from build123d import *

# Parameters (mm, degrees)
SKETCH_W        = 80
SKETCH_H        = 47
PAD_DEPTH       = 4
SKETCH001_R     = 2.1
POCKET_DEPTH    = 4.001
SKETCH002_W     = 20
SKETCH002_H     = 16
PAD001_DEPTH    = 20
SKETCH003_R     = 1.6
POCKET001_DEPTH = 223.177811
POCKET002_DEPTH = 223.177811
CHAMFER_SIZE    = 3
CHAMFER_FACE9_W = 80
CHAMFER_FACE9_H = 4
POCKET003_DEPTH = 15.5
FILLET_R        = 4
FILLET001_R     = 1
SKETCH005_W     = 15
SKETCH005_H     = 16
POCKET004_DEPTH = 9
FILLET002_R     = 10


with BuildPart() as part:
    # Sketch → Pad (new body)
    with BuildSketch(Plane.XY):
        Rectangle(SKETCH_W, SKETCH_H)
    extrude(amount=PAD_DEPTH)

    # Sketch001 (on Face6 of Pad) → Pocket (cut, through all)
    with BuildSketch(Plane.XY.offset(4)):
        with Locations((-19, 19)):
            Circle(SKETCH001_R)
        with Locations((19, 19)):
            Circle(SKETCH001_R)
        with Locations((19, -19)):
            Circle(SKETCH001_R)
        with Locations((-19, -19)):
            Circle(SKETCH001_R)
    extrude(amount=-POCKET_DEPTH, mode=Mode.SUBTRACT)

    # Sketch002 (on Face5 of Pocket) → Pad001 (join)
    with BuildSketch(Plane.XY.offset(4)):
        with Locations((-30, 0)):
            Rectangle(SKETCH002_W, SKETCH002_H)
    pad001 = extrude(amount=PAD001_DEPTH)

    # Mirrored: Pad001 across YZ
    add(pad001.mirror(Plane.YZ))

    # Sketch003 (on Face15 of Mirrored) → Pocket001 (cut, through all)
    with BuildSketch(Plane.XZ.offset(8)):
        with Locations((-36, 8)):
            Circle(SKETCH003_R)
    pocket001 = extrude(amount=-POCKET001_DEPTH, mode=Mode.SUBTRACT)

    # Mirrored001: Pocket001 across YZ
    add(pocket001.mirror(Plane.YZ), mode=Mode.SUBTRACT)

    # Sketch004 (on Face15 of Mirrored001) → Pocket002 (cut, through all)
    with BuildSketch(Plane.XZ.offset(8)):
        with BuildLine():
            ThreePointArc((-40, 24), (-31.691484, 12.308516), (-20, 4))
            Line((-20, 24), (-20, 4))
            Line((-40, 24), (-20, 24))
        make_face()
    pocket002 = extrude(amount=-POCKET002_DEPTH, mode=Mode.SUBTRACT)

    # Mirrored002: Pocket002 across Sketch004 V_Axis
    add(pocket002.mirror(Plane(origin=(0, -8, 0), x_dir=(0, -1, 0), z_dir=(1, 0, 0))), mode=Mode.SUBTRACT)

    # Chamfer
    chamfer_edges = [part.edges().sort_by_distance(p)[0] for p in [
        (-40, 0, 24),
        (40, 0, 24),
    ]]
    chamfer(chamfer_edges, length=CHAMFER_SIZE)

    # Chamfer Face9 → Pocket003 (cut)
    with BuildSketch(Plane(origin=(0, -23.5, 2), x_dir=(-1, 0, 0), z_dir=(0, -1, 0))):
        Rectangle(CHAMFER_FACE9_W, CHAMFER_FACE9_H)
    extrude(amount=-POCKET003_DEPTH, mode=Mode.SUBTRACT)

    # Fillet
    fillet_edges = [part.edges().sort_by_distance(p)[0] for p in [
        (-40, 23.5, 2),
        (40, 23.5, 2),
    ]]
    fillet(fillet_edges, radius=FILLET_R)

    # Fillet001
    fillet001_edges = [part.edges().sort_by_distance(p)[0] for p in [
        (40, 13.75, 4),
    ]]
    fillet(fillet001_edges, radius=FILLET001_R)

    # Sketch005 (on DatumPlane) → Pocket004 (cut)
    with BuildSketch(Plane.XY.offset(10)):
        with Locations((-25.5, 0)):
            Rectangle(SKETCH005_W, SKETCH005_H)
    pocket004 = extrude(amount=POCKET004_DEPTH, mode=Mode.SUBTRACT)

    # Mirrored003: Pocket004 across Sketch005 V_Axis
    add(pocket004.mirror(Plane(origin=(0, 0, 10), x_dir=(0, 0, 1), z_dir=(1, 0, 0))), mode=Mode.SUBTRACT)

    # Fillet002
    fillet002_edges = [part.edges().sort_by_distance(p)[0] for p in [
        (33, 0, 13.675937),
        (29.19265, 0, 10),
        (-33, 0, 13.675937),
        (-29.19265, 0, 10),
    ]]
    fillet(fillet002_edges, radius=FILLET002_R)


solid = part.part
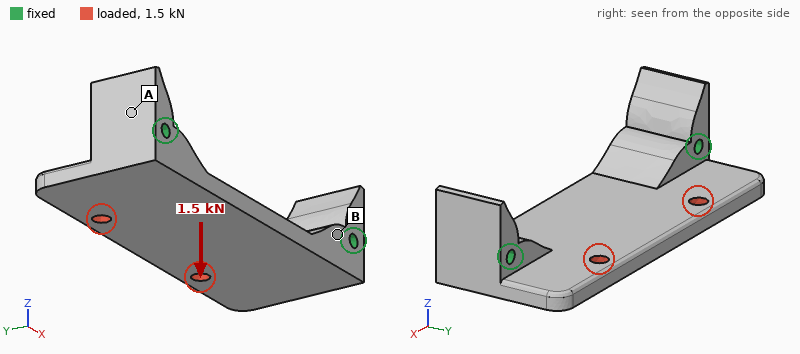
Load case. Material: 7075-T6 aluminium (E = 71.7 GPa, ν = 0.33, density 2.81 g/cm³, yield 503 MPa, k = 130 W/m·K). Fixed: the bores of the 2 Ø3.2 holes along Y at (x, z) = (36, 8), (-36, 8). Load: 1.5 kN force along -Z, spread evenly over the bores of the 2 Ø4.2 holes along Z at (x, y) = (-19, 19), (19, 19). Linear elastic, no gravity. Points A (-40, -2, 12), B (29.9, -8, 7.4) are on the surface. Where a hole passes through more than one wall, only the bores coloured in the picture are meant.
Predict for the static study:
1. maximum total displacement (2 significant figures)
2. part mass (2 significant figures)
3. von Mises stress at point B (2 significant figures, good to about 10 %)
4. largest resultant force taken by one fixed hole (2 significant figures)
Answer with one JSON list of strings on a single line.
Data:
["0.20 mm", "40 g", "23 MPa", "1.2 kN"]
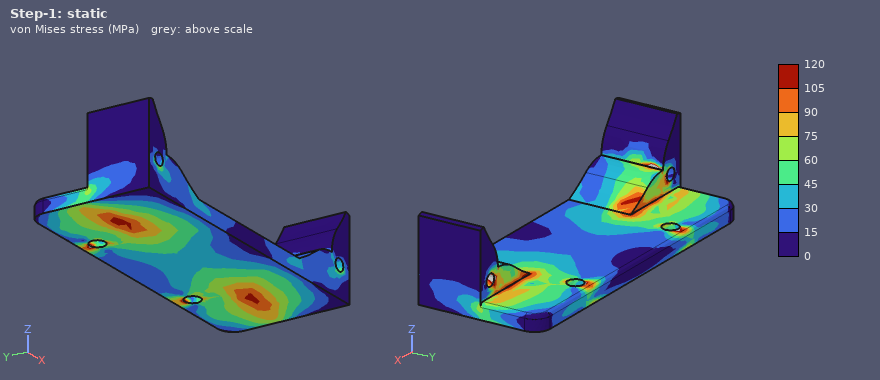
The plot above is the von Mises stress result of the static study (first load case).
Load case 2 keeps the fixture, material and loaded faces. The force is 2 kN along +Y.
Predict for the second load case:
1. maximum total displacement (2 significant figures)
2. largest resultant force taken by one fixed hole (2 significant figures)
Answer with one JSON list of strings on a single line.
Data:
["17 µm", "1.0 kN"]
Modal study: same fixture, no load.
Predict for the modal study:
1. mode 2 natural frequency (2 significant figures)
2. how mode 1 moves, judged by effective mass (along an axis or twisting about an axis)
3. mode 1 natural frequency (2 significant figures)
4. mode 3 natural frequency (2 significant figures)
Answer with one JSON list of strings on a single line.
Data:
["8700 Hz", "along Z", "5200 Hz", "9200 Hz"]
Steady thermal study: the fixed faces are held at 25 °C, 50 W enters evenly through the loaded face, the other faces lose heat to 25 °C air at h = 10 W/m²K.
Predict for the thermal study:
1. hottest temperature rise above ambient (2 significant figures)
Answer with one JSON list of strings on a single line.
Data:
["50 K"]
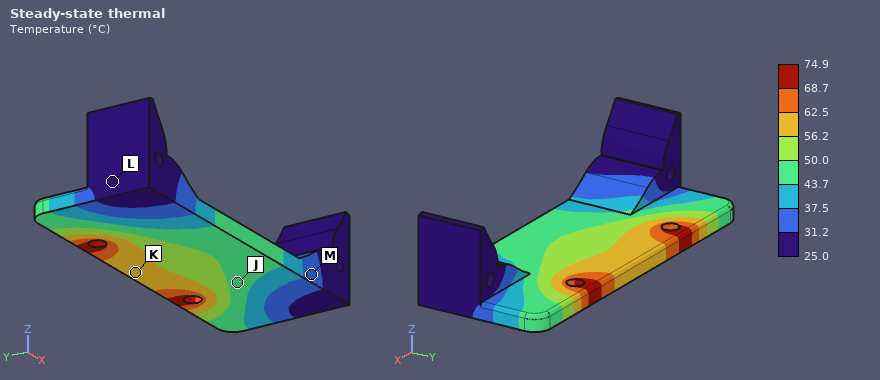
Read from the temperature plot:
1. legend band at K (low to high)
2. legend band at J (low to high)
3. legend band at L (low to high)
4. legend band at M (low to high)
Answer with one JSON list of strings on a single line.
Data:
["56.2 to 62.5 °C", "43.7 to 50.0 °C", "25.0 to 31.2 °C", "31.2 to 37.5 °C"]
